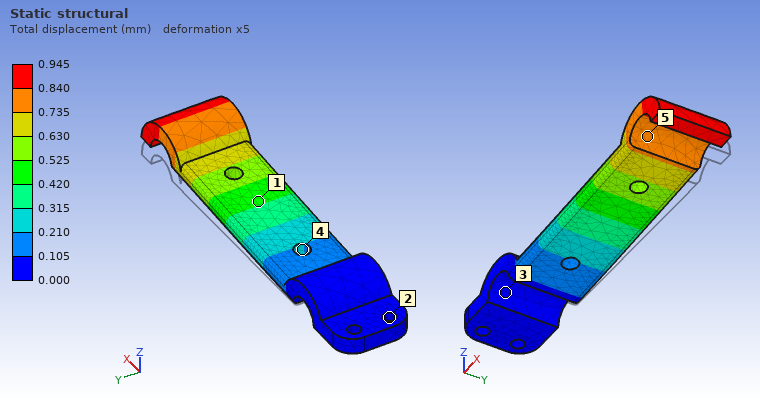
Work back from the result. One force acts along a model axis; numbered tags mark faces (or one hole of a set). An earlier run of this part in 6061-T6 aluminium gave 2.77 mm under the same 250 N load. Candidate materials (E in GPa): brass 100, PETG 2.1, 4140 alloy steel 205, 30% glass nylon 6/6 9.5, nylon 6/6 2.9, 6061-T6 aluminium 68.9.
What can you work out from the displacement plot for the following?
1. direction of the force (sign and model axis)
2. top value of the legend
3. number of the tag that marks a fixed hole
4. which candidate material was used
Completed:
+Z
0.945 mm
2
4140 alloy steel
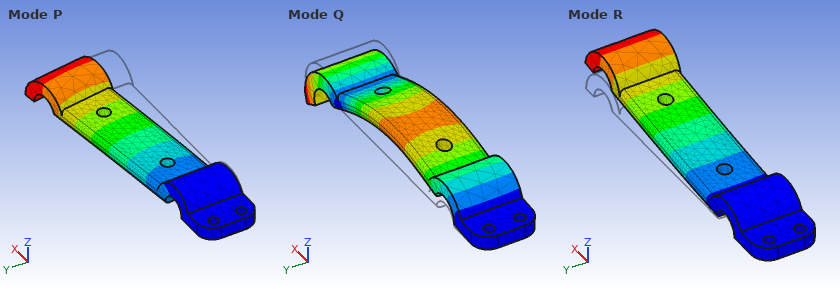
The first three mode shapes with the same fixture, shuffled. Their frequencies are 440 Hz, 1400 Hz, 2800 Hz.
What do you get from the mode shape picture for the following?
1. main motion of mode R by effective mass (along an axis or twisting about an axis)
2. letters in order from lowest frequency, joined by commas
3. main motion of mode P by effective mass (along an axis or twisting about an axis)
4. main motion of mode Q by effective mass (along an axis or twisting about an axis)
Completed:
along Z
R, P, Q
along Y
along Z
